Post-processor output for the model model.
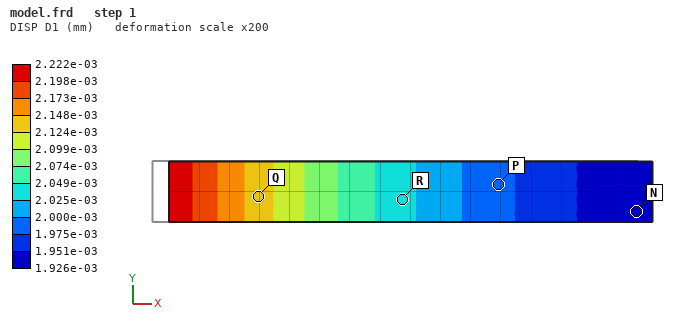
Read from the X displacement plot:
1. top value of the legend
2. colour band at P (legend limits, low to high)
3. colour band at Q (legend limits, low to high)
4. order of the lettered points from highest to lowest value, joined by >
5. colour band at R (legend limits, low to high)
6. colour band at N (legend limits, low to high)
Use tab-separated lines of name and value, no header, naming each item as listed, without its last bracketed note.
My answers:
top value of the legend	2.222e-03 mm
colour band at P	1.975e-03 to 2.000e-03 mm
colour band at Q	2.124e-03 to 2.148e-03 mm
order of the lettered points from highest to lowest value, joined by >	Q > R > P > N
colour band at R	2.025e-03 to 2.049e-03 mm
colour band at N	1.926e-03 to 1.951e-03 mm
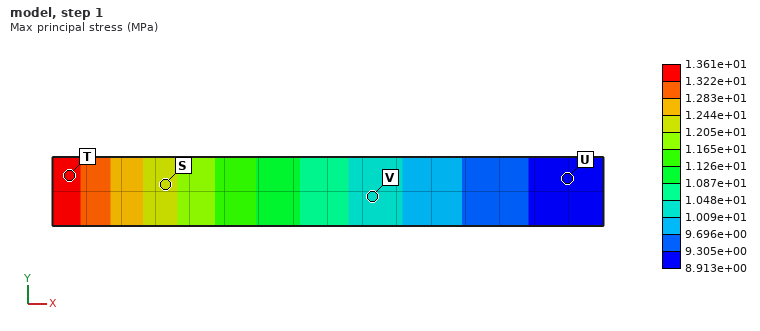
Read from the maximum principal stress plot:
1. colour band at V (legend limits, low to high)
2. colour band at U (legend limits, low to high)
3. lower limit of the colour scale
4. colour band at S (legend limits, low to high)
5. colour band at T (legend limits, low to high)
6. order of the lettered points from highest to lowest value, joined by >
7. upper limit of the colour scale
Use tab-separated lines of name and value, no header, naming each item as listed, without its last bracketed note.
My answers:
colour band at V	1.009e+01 to 1.048e+01 MPa
colour band at U	8.913e+00 to 9.305e+00 MPa
lower limit of the colour scale	8.913e+00 MPa
colour band at S	1.205e+01 to 1.244e+01 MPa
colour band at T	1.322e+01 to 1.361e+01 MPa
order of the lettered points from highest to lowest value, joined by >	T > S > V > U
upper limit of the colour scale	1.361e+01 MPa
